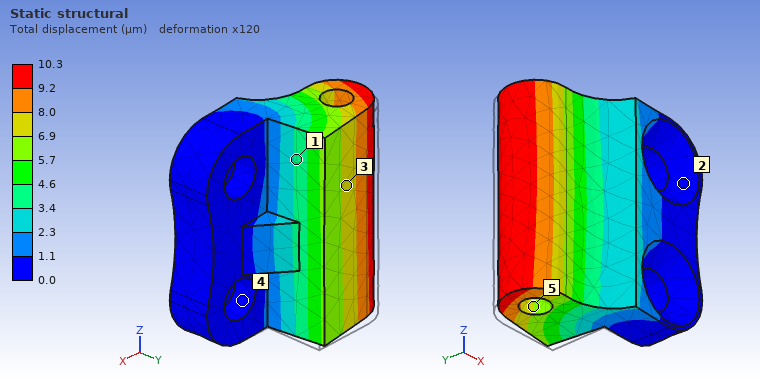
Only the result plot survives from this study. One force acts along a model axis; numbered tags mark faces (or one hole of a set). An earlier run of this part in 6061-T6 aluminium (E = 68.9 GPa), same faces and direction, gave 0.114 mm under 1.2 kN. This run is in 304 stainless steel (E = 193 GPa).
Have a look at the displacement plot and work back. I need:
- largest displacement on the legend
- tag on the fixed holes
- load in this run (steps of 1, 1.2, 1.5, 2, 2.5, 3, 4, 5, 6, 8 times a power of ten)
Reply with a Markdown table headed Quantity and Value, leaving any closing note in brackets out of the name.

| Quantity | Value |
|---|---|
| largest displacement on the legend | 10.3 µm |
| tag on the fixed holes | 4 |
| load in this run | 300 N |
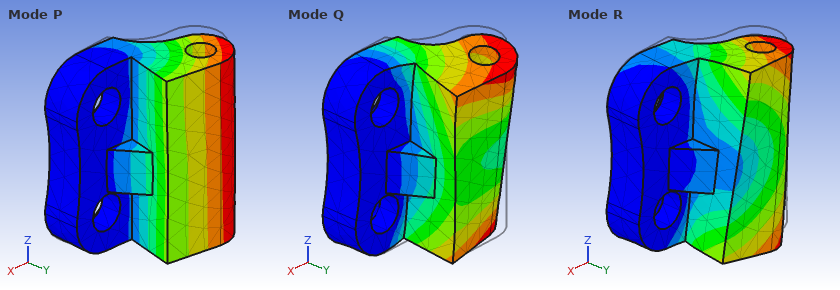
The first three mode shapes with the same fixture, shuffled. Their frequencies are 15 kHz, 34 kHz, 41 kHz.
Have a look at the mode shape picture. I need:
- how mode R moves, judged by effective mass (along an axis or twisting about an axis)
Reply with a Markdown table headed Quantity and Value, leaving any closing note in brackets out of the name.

| Quantity | Value |
|---|---|
| how mode R moves, judged by effective mass | along Z |
